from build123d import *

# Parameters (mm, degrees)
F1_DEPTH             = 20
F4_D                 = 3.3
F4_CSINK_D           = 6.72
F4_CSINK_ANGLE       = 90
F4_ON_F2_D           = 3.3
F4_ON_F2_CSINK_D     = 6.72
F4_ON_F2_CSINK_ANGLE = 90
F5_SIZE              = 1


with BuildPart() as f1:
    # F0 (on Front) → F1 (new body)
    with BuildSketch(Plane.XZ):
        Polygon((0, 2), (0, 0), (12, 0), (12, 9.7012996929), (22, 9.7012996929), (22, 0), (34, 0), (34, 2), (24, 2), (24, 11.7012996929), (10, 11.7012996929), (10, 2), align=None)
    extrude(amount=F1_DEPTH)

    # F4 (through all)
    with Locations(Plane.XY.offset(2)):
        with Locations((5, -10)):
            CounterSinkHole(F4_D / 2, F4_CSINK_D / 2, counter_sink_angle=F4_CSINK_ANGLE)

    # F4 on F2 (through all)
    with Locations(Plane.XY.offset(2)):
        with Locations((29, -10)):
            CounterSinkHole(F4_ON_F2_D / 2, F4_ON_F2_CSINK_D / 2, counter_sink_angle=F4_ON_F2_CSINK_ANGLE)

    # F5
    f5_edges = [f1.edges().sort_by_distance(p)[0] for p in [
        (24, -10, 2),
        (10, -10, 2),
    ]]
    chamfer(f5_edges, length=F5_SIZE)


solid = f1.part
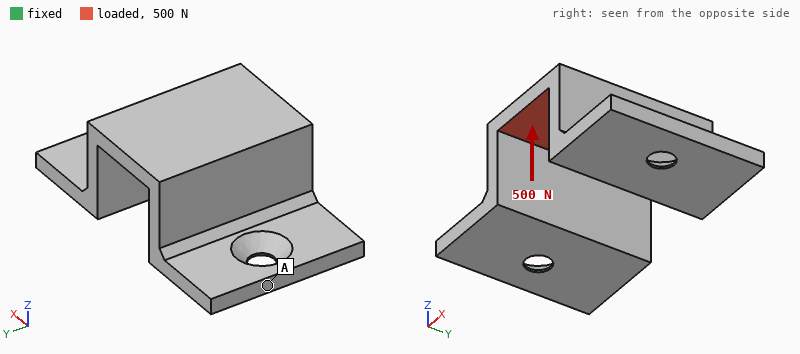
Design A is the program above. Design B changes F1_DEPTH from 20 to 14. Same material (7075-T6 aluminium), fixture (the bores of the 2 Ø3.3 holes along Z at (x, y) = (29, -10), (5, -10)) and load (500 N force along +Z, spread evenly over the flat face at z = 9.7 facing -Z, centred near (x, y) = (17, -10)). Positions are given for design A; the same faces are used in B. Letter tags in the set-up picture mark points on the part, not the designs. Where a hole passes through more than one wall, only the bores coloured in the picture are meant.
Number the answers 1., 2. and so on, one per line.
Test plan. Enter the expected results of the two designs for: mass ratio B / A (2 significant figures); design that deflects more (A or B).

1. 0.69
2. B
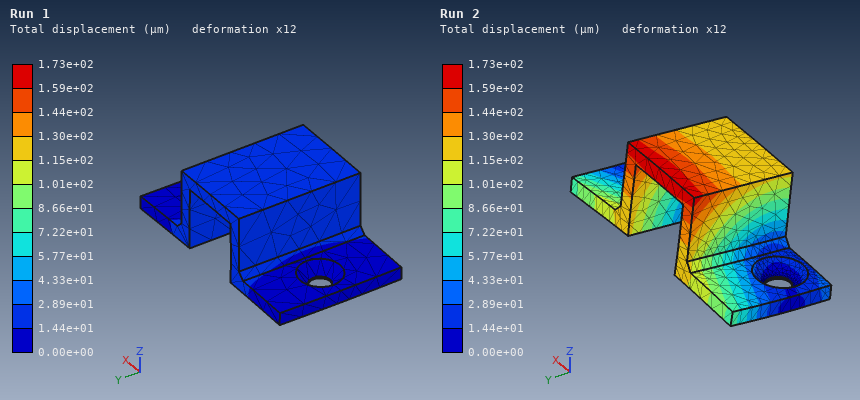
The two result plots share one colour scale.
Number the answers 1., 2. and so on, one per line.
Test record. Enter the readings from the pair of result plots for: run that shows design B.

1. Run 2
